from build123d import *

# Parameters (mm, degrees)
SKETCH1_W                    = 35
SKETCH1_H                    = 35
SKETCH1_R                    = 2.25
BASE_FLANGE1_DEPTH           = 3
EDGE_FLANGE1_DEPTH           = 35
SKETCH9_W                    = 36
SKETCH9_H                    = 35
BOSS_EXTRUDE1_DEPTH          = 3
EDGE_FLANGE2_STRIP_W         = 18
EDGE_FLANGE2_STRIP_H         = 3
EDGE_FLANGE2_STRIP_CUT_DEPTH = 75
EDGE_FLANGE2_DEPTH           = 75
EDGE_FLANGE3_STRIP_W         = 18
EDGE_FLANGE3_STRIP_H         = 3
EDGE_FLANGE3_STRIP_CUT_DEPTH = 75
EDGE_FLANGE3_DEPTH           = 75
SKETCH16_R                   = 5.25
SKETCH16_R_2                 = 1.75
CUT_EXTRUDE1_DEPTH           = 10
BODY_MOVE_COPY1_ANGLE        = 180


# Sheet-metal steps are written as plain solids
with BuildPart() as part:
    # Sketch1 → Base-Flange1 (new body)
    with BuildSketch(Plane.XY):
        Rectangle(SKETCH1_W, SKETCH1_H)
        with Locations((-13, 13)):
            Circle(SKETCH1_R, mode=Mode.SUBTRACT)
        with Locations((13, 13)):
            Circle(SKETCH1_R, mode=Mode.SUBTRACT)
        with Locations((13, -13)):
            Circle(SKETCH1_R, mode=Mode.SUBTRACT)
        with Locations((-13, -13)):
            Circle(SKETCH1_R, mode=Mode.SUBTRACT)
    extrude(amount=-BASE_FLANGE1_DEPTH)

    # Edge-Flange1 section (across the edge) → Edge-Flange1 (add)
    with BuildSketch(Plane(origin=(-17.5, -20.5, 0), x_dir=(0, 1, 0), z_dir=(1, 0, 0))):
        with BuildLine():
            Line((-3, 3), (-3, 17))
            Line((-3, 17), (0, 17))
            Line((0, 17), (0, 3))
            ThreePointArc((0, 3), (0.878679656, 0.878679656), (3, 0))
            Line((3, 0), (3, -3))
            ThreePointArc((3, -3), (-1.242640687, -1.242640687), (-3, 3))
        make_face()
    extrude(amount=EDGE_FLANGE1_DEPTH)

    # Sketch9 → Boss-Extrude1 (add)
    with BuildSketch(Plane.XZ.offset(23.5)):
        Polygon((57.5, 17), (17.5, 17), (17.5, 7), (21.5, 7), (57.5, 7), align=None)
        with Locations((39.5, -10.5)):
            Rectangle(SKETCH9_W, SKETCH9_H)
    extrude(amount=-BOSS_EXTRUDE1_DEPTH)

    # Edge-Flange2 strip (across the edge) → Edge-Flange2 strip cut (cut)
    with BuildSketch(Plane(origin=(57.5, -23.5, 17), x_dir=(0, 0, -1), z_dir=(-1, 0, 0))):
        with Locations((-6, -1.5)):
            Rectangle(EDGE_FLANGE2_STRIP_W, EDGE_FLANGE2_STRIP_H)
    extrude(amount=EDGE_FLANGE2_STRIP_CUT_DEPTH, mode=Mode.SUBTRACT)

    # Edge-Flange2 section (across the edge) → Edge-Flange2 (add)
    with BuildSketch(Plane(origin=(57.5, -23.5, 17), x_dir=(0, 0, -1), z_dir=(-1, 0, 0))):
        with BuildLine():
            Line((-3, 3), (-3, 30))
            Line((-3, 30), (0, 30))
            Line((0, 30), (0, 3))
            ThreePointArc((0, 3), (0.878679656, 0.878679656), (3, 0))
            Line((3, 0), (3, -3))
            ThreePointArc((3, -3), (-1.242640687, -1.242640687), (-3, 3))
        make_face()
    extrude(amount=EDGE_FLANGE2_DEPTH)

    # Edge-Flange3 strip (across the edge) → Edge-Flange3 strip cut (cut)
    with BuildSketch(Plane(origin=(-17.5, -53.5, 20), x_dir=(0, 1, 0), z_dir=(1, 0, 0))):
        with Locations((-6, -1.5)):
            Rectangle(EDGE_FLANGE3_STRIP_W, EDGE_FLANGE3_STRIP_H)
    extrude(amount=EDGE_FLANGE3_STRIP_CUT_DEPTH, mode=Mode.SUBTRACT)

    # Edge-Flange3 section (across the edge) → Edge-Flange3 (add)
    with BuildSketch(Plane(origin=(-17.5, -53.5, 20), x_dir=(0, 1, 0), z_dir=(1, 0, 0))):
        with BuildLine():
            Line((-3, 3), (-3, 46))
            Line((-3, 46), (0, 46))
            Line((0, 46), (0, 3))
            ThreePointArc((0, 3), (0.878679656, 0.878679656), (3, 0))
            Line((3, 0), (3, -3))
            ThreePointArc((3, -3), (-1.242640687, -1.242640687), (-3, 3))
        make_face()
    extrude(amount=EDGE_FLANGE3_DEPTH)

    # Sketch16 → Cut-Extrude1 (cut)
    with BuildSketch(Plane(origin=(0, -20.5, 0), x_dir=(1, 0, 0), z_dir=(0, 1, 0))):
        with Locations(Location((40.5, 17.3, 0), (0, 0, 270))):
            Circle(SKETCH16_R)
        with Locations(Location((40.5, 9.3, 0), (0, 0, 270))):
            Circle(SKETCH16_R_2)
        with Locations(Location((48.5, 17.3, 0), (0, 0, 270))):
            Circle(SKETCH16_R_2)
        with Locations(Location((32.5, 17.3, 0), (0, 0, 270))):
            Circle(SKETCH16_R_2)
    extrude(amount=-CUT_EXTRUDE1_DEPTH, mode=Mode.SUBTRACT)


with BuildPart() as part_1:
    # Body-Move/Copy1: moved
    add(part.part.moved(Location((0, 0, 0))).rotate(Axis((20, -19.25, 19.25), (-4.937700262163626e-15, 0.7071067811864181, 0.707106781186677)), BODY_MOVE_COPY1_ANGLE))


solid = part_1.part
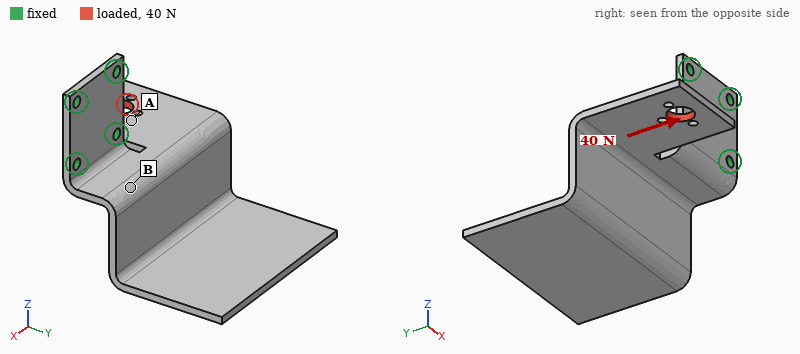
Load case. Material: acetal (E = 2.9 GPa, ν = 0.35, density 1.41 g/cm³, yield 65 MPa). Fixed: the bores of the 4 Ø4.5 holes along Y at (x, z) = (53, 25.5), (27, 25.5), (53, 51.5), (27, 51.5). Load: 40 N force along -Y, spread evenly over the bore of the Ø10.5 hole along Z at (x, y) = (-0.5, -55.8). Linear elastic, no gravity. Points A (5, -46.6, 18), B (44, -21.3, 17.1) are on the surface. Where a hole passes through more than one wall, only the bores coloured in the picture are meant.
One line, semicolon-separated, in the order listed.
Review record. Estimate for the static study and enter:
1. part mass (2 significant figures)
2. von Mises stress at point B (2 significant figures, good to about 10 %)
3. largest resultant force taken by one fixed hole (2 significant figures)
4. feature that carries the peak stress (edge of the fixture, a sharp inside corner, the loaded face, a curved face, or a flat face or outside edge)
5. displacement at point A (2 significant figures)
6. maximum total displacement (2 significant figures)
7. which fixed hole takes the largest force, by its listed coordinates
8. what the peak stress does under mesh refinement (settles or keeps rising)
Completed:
39 g; 2.7 MPa; 83 N; edge of the fixture; 0.51 mm; 1.4 mm; (27, 25.5); keeps rising
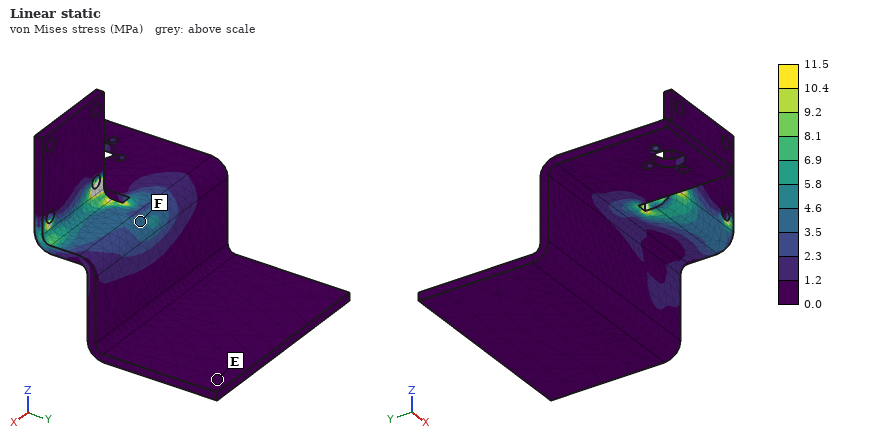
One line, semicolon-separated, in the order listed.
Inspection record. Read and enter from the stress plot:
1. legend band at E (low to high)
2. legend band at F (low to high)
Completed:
0.0 to 1.2 MPa; 3.5 to 4.6 MPa
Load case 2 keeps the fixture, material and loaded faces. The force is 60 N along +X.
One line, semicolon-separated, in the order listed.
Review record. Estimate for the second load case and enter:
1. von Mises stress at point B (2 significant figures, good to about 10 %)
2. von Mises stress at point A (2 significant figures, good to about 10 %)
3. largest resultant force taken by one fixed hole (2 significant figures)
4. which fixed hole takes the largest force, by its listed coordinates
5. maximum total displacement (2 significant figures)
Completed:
3.3 MPa; 1.5 MPa; 55 N; (27, 25.5); 1.4 mm
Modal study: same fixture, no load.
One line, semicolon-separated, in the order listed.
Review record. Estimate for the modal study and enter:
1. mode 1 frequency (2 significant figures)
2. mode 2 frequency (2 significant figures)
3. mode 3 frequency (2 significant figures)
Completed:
62 Hz; 160 Hz; 200 Hz
